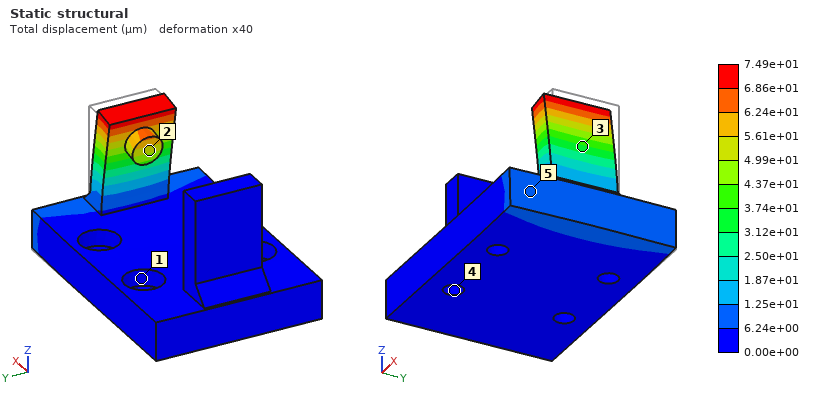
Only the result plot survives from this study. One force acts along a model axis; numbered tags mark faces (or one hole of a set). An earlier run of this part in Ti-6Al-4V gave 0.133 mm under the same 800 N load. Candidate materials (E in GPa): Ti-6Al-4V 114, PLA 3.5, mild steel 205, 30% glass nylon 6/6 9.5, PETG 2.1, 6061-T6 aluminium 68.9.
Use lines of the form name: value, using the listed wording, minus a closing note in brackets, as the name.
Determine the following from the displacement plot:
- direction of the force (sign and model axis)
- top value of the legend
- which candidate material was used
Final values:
direction of the force: -X
top value of the legend: 7.49e+01 µm
which candidate material was used: mild steel
